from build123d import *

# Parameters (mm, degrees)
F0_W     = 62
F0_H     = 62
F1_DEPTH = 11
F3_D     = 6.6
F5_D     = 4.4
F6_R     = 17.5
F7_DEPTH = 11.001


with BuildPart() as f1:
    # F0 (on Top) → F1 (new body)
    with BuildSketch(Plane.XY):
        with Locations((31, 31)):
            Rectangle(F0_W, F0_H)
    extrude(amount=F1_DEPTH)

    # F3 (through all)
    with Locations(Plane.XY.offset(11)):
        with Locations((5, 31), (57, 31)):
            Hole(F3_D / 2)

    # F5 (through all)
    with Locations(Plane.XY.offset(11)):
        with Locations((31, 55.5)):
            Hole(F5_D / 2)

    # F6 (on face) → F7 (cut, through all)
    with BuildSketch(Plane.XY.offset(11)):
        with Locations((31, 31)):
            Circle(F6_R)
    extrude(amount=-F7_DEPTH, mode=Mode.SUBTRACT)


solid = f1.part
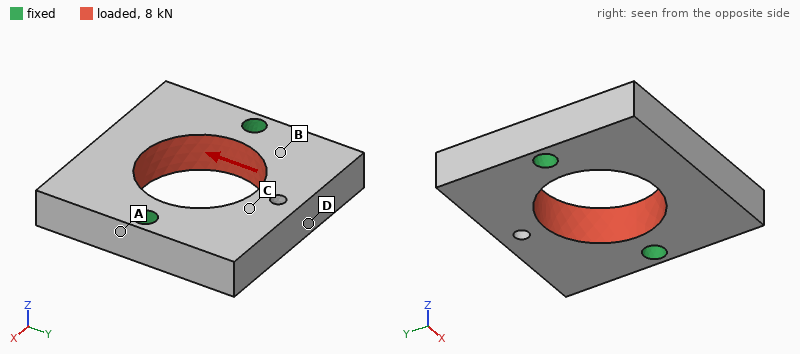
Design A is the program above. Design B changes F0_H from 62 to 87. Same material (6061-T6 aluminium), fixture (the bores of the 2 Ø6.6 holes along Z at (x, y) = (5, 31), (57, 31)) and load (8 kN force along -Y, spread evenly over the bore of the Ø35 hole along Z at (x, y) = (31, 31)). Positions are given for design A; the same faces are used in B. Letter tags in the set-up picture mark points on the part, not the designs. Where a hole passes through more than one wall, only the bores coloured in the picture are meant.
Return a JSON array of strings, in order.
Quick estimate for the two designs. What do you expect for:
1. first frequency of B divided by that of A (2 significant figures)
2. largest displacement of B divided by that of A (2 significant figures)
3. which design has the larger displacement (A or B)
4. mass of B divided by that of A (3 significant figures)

["0.54", "0.69", "A", "1.55"]
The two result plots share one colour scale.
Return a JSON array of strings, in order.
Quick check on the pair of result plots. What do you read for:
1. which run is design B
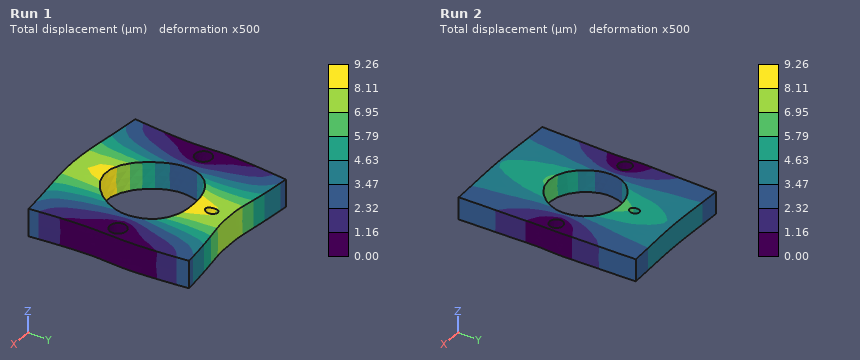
["Run 2"]
